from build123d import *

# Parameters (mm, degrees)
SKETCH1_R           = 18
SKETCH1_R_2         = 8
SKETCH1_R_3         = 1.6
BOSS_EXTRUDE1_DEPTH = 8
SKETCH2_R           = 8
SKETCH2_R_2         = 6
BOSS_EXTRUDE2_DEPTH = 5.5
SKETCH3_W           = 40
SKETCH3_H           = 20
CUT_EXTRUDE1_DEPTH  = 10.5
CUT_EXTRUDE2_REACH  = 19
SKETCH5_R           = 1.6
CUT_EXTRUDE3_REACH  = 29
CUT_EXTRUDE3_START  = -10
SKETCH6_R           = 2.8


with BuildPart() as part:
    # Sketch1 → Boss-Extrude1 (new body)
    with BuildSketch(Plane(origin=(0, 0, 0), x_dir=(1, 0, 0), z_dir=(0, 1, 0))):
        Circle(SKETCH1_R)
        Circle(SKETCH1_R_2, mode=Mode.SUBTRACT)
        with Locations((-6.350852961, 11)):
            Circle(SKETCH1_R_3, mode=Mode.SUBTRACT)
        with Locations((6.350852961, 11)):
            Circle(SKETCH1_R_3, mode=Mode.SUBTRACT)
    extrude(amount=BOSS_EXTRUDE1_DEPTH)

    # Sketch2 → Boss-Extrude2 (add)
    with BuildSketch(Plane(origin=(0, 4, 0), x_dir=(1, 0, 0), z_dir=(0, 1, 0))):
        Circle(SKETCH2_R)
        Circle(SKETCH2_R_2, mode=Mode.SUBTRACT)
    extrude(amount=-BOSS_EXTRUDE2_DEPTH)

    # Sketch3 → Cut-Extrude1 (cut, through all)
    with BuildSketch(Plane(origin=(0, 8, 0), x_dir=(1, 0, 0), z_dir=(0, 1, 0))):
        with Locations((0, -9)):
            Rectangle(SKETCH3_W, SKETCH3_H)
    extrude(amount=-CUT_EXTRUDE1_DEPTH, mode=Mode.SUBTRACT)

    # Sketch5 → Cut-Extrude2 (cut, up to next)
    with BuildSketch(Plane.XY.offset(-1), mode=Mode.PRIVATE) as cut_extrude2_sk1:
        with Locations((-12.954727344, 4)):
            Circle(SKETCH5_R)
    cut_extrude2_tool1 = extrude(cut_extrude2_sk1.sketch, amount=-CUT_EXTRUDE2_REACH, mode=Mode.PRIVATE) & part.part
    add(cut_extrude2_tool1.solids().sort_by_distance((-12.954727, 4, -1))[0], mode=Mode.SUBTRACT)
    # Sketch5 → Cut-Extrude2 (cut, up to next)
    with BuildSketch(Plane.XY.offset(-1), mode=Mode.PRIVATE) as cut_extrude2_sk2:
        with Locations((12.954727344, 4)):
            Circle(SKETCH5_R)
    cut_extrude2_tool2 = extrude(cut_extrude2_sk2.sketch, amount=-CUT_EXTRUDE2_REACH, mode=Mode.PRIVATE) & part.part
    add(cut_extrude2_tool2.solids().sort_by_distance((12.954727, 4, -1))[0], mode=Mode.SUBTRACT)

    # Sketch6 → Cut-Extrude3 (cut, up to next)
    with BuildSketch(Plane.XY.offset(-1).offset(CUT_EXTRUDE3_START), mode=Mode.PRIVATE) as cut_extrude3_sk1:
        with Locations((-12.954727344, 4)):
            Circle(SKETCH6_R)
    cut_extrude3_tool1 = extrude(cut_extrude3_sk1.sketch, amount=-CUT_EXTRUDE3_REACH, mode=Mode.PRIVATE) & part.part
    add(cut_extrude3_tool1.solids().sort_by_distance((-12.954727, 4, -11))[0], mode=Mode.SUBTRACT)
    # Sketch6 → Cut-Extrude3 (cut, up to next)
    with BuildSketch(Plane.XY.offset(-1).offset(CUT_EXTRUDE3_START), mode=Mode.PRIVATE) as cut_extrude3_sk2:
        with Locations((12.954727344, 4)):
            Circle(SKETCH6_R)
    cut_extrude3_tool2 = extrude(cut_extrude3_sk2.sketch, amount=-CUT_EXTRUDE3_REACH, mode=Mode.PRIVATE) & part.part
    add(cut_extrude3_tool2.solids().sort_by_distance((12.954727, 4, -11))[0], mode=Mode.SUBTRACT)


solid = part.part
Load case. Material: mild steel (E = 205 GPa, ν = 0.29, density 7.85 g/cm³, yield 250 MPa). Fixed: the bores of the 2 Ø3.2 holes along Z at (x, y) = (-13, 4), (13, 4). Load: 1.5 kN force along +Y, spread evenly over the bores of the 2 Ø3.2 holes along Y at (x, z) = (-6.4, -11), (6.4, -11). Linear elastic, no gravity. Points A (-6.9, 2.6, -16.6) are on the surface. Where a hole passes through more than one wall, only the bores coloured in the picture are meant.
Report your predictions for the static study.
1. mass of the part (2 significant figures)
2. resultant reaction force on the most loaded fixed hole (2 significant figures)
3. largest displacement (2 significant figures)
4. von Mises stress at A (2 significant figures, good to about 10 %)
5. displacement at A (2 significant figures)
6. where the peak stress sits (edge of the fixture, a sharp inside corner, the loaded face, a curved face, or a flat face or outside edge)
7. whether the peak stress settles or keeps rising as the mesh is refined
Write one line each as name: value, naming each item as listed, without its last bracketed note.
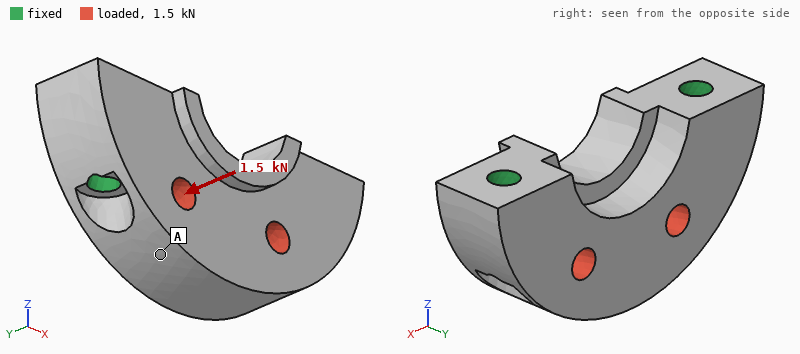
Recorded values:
mass of the part: 23 g
resultant reaction force on the most loaded fixed hole: 750 N
largest displacement: 4.4 µm
von Mises stress at A: 11 MPa
displacement at A: 3.6 µm
where the peak stress sits: edge of the fixture
whether the peak stress settles or keeps rising as the mesh is refined: keeps rising
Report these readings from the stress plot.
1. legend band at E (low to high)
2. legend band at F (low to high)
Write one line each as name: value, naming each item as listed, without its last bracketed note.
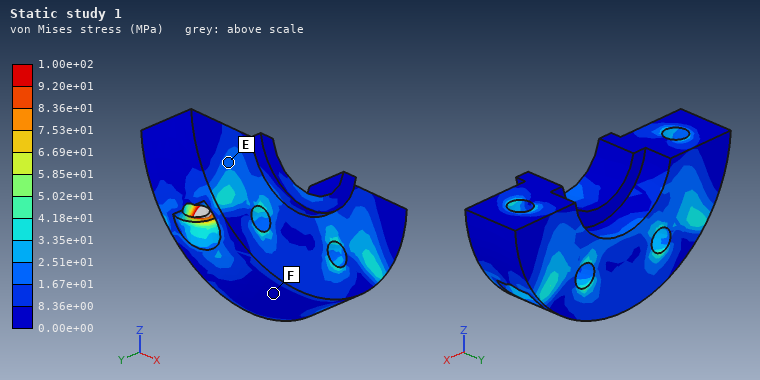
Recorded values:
legend band at E: 1.67e+01 to 2.51e+01 MPa
legend band at F: 0.00e+00 to 8.36e+00 MPa
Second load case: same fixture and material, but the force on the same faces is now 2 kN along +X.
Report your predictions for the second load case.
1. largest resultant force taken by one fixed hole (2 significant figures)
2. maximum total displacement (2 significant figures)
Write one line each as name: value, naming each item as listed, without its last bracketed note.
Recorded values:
largest resultant force taken by one fixed hole: 1.0 kN
maximum total displacement: 1.0 µm
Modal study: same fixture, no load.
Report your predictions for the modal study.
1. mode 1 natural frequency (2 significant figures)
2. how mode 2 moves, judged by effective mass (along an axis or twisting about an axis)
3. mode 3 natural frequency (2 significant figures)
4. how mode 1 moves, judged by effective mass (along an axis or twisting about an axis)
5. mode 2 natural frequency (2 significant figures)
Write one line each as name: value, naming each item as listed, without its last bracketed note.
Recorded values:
mode 1 natural frequency: 27 kHz
how mode 2 moves, judged by effective mass: along Z
mode 3 natural frequency: 55 kHz
how mode 1 moves, judged by effective mass: along Y
mode 2 natural frequency: 49 kHz
